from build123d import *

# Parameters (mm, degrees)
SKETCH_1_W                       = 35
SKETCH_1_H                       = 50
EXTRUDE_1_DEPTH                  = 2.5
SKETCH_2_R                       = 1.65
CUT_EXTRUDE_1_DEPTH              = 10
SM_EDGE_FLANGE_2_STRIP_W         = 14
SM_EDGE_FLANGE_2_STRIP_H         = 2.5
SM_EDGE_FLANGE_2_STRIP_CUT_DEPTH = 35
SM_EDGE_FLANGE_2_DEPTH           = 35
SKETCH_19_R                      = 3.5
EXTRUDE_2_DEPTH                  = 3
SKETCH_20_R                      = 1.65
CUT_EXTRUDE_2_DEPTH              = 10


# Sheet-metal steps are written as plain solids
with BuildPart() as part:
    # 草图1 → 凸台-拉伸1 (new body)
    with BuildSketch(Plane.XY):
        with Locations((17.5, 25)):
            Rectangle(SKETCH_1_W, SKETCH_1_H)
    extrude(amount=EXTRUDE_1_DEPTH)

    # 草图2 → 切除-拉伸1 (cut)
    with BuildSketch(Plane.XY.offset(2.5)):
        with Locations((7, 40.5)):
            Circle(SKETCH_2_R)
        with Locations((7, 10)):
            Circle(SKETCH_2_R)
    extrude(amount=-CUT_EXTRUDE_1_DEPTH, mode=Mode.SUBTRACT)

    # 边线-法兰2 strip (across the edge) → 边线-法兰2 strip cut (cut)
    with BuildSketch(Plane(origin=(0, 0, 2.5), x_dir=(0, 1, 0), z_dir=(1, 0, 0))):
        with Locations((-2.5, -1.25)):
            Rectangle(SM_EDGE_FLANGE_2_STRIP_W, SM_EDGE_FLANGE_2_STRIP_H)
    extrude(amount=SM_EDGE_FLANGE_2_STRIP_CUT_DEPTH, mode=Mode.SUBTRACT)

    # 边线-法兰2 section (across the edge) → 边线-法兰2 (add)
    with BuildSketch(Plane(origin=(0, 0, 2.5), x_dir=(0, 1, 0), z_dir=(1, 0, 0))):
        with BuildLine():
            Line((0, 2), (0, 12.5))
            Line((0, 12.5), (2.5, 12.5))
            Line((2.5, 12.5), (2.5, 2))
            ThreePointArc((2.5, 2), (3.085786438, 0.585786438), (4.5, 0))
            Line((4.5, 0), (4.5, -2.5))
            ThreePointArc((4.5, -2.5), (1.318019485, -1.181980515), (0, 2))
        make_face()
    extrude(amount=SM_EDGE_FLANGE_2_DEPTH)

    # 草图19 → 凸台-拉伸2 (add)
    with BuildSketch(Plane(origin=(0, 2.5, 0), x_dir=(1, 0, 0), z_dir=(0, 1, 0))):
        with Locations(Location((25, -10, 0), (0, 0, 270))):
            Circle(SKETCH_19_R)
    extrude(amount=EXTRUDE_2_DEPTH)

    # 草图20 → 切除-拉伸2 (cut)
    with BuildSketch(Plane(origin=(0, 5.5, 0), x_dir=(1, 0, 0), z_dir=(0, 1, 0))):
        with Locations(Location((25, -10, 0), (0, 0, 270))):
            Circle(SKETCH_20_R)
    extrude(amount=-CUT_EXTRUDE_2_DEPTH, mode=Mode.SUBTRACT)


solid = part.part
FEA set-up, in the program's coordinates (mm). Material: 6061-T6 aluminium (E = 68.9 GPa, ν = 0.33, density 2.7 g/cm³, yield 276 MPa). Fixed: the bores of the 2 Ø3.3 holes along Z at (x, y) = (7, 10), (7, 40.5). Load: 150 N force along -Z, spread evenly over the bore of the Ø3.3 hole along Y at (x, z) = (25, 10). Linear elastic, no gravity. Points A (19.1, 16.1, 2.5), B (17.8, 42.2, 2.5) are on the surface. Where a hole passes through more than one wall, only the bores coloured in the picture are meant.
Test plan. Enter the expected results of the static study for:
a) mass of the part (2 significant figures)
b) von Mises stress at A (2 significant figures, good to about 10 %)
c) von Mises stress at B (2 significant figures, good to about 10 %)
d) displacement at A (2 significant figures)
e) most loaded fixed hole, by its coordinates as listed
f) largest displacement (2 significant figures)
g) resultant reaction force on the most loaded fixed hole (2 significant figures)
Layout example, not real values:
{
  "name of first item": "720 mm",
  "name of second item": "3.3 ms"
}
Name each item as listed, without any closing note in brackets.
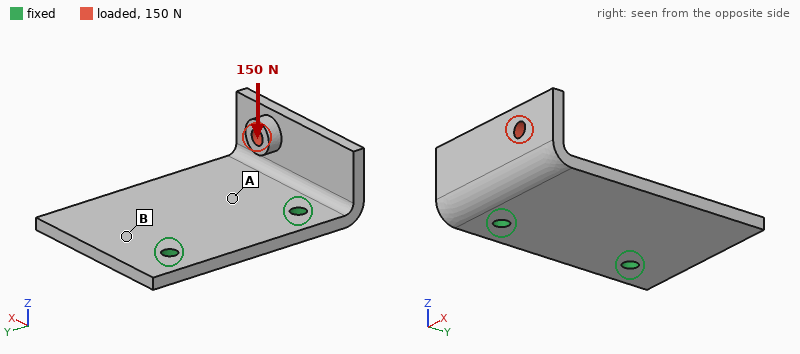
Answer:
{
  "mass of the part": "15 g",
  "von Mises stress at A": "28 MPa",
  "von Mises stress at B": "9.9 MPa",
  "displacement at A": "0.034 mm",
  "most loaded fixed hole, by its coordinates as listed": "(7, 10)",
  "largest displacement": "0.20 mm",
  "resultant reaction force on the most loaded fixed hole": "160 N"
}
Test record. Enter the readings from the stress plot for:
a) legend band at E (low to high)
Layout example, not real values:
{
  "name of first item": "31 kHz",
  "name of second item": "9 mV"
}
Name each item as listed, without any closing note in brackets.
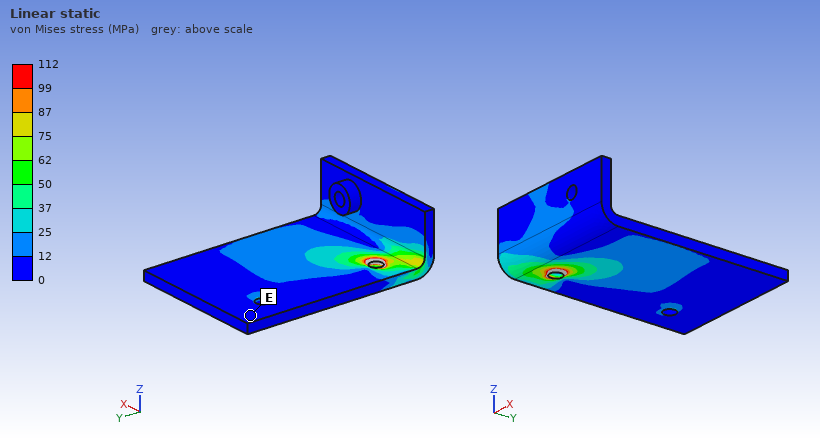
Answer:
{
  "legend band at E": "0 to 12 MPa"
}
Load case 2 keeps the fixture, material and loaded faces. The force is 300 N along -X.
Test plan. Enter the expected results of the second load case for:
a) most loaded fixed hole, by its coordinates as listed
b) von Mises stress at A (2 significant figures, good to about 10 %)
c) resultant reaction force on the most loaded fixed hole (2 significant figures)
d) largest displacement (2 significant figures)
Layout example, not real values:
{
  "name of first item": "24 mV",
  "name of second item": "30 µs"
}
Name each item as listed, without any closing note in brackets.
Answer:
{
  "most loaded fixed hole, by its coordinates as listed": "(7, 10)",
  "von Mises stress at A": "25 MPa",
  "resultant reaction force on the most loaded fixed hole": "360 N",
  "largest displacement": "0.20 mm"
}
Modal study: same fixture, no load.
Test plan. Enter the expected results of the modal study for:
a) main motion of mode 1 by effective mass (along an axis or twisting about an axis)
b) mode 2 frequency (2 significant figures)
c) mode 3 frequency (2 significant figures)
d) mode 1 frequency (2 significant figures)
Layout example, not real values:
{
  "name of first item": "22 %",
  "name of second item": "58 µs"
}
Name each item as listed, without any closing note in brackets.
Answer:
{
  "main motion of mode 1 by effective mass": "along Z",
  "mode 2 frequency": "3300 Hz",
  "mode 3 frequency": "5200 Hz",
  "mode 1 frequency": "2500 Hz"
}
